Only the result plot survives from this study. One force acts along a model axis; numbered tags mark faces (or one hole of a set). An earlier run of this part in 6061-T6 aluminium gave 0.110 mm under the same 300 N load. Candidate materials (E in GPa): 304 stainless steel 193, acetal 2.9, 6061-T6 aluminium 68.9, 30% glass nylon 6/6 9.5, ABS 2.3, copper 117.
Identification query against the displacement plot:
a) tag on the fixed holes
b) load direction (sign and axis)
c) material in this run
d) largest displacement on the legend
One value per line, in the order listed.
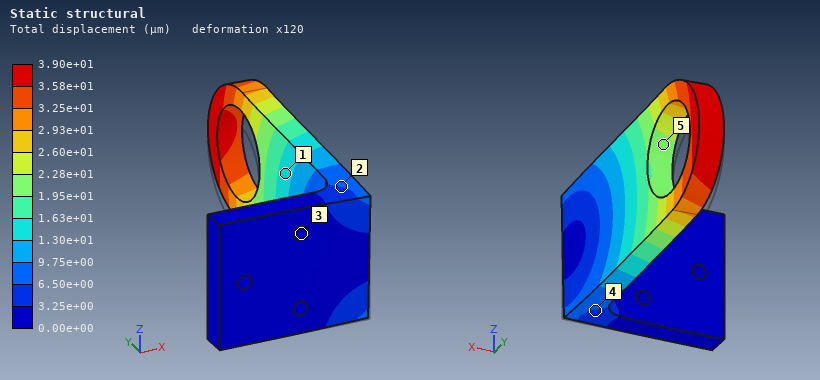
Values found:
3
+Z
304 stainless steel
3.90e+01 µm
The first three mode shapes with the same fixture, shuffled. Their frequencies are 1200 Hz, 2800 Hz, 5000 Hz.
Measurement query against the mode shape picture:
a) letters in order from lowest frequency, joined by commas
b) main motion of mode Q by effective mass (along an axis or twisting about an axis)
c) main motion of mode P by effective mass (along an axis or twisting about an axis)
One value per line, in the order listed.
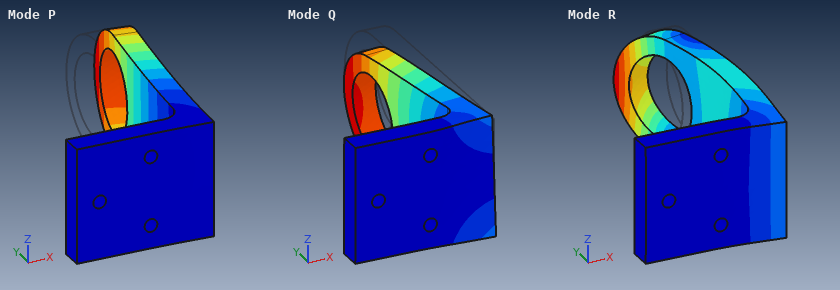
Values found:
P, Q, R
along Z
along X
